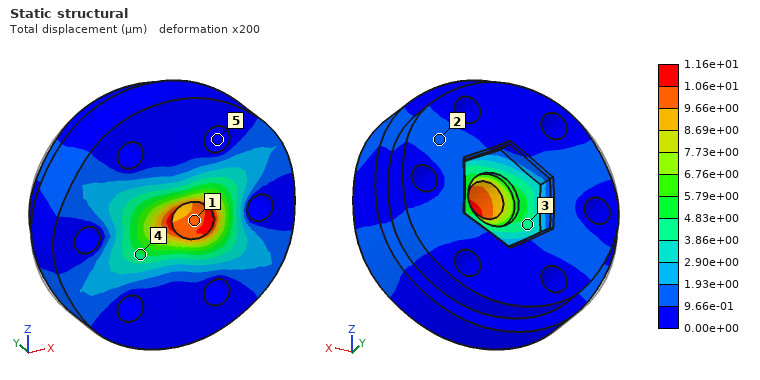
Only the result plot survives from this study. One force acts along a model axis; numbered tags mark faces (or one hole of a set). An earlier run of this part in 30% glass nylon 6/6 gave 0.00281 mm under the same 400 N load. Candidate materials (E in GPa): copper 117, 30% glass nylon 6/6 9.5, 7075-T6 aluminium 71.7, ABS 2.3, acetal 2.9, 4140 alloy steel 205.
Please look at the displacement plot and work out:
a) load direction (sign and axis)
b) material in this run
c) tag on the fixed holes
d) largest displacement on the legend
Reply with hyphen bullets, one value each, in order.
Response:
- +X
- ABS
- 5
- 1.16e+01 µm
